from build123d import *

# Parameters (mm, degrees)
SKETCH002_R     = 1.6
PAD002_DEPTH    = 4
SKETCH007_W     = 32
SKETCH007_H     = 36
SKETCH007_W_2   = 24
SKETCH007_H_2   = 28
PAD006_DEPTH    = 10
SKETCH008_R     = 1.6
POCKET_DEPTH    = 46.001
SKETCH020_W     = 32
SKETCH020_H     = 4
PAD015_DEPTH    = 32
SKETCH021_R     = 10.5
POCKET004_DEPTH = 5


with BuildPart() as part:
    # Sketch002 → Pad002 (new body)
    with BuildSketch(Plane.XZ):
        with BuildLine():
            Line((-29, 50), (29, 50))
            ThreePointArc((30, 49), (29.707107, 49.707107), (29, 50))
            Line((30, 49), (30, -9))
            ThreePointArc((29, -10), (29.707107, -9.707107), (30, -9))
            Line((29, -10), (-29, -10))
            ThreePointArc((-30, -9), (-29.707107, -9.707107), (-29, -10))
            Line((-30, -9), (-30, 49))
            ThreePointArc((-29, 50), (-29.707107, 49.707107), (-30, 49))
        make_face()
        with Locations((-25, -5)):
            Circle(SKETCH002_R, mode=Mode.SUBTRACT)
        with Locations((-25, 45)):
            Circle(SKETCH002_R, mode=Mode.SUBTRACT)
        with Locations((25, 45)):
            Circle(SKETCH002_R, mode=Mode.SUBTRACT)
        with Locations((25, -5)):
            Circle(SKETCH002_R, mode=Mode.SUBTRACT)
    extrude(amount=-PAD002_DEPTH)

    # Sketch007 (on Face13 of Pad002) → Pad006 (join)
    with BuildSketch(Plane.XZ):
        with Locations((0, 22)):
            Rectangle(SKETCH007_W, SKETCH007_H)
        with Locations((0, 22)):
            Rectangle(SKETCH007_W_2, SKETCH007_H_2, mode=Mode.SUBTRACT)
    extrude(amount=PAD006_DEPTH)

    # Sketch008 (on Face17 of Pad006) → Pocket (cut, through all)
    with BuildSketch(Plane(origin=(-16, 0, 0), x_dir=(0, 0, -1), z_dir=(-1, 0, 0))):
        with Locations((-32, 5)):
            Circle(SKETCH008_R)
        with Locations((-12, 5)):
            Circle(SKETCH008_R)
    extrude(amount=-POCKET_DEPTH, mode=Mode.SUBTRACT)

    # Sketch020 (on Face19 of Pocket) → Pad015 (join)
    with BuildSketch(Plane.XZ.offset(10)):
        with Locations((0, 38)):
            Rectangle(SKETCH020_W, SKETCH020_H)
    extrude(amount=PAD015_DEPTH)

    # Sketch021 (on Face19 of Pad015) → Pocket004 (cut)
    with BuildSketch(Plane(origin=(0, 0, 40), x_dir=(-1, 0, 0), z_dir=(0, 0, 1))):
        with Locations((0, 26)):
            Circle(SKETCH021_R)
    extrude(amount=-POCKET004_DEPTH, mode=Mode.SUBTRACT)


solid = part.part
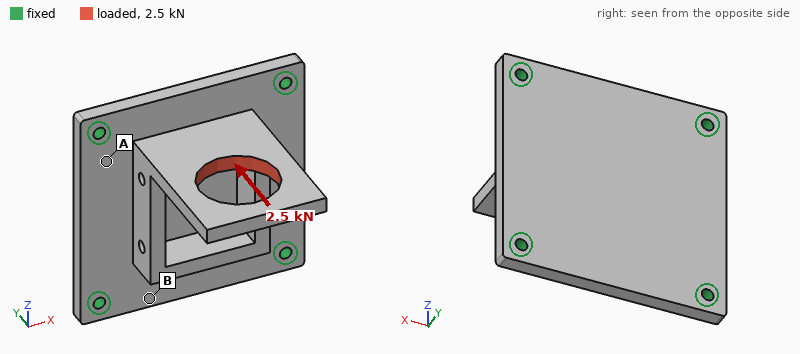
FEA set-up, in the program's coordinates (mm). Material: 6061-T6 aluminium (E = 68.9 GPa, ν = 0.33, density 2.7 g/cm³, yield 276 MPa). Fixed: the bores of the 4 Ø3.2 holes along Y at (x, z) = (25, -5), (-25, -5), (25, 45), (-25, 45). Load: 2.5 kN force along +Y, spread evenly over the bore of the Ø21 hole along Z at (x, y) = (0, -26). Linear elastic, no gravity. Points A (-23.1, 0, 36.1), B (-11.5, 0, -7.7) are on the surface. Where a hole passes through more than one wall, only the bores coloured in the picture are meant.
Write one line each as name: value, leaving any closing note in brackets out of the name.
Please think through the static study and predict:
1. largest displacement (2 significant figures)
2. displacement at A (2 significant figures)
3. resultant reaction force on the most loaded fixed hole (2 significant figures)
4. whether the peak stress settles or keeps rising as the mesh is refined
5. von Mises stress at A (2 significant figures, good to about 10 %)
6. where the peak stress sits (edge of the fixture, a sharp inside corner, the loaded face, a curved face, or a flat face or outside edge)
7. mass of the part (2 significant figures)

largest displacement: 0.11 mm
displacement at A: 0.023 mm
resultant reaction force on the most loaded fixed hole: 1.2 kN
whether the peak stress settles or keeps rising as the mesh is refined: keeps rising
von Mises stress at A: 30 MPa
where the peak stress sits: edge of the fixture
mass of the part: 58 g
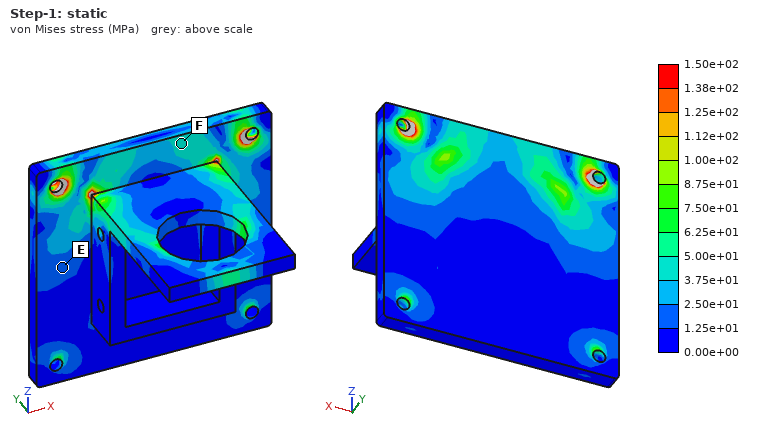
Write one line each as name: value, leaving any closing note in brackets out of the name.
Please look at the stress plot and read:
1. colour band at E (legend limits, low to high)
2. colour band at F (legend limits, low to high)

colour band at E: 1.25e+01 to 2.50e+01 MPa
colour band at F: 3.75e+01 to 5.00e+01 MPa
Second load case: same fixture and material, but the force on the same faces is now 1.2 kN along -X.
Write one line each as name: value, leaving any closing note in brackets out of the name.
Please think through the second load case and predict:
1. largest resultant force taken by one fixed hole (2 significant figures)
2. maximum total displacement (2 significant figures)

largest resultant force taken by one fixed hole: 840 N
maximum total displacement: 0.15 mm
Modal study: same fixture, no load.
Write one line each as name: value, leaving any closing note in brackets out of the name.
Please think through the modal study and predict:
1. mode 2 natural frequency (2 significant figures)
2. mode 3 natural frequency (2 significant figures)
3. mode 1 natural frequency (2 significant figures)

mode 2 natural frequency: 5200 Hz
mode 3 natural frequency: 5700 Hz
mode 1 natural frequency: 2200 Hz
